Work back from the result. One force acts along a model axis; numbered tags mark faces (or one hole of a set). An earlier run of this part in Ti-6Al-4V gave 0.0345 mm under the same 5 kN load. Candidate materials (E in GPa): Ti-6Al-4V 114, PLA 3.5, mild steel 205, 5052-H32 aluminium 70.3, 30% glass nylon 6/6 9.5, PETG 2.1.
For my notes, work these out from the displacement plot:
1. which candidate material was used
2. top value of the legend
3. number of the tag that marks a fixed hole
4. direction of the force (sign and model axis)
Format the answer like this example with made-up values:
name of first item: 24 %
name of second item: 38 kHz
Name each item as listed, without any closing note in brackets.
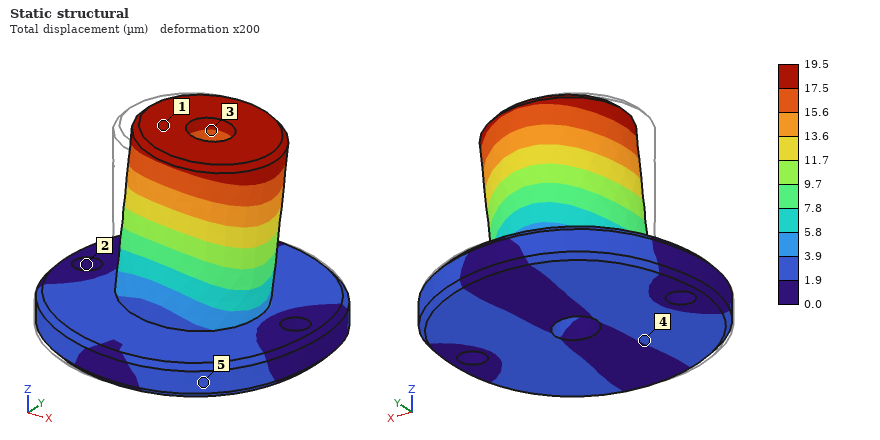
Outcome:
which candidate material was used: mild steel
top value of the legend: 19.5 µm
number of the tag that marks a fixed hole: 2
direction of the force: +X
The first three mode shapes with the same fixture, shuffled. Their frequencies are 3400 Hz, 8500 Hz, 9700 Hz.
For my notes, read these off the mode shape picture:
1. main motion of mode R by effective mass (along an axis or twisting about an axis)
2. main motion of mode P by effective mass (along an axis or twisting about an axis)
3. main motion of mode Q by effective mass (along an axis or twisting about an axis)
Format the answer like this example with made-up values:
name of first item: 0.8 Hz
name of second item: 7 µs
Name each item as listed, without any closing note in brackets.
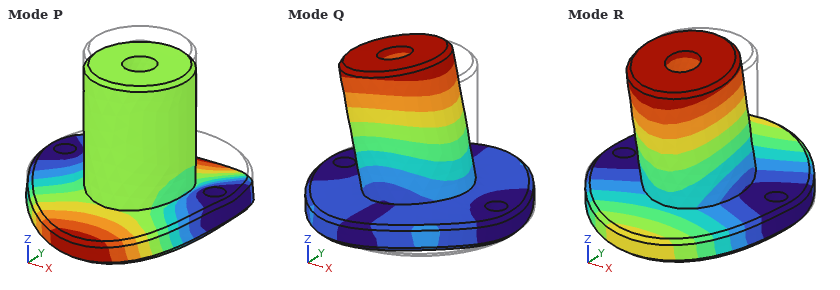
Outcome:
main motion of mode R by effective mass: along Y
main motion of mode P by effective mass: along Z
main motion of mode Q by effective mass: along X
